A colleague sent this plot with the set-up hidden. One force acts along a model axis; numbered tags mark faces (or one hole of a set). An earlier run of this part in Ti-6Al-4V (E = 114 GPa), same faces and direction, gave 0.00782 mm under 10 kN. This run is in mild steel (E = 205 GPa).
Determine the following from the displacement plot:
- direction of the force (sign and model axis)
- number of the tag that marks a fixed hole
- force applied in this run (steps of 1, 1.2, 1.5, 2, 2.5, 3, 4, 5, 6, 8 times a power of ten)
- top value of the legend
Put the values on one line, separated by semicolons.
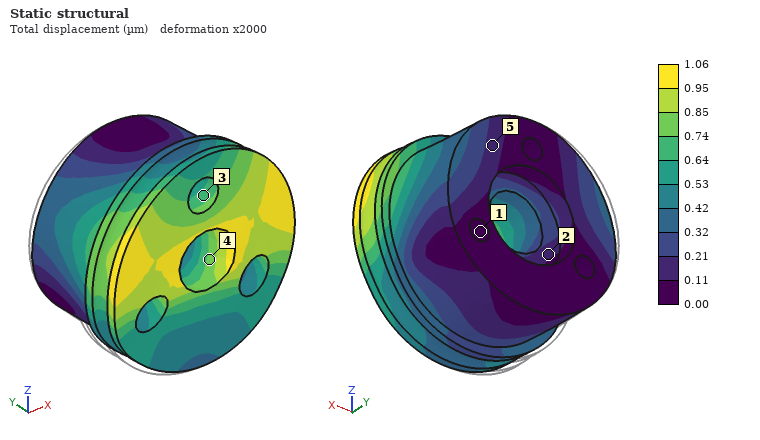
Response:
+X; 1; 2.5 kN; 1.06 µm
